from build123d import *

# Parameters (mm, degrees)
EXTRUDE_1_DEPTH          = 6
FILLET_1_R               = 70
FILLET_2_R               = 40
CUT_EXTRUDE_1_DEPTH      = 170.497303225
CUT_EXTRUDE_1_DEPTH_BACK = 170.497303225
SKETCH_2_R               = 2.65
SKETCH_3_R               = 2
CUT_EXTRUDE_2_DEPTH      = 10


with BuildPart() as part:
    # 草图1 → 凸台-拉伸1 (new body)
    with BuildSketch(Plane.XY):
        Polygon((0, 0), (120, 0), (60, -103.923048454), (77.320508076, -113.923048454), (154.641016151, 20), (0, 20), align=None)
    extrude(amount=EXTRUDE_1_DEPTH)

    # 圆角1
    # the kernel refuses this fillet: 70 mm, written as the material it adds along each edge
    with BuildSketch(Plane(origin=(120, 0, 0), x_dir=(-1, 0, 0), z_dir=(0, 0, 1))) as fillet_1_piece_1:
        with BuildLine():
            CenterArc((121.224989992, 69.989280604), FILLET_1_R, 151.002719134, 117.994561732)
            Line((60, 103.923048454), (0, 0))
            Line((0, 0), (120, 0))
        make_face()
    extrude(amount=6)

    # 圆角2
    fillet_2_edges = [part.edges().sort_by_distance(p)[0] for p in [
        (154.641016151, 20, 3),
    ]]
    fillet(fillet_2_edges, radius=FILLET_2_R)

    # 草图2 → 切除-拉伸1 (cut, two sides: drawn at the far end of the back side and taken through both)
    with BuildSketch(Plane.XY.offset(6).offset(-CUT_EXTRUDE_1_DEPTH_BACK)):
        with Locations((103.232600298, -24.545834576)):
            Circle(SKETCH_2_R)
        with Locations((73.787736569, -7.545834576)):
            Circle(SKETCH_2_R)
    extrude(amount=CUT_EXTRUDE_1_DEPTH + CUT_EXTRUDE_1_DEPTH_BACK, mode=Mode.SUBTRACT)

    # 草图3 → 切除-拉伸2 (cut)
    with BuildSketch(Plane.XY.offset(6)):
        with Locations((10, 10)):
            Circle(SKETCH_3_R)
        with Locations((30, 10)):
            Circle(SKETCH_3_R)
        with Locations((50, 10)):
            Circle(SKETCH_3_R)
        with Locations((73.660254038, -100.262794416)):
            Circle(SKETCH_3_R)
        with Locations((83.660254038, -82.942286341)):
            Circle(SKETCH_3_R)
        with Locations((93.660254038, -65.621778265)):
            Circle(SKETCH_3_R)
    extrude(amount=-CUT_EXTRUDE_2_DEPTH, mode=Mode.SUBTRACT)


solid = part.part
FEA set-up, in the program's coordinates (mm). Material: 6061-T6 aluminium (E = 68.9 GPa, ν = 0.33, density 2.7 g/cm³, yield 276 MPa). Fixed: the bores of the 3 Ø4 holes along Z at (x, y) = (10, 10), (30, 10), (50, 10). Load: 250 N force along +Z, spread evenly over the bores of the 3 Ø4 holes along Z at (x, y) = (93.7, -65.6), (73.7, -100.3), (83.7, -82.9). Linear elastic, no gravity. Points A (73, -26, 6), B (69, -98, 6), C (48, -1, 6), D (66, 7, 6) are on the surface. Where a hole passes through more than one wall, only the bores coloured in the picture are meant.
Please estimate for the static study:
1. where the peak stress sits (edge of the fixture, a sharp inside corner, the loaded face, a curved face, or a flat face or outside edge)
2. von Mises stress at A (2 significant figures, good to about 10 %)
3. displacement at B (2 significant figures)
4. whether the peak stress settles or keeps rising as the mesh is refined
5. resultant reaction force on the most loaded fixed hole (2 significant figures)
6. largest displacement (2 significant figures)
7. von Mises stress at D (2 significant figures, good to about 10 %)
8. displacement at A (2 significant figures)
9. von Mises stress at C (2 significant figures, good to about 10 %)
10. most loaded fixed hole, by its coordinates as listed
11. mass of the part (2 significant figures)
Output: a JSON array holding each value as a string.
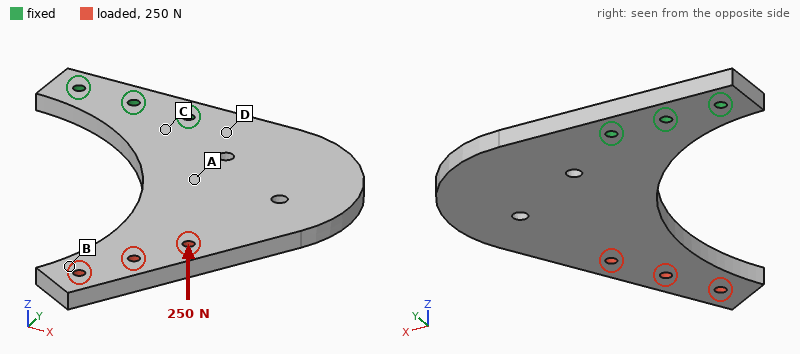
["edge of the fixture", "44 MPa", "1.8 mm", "keeps rising", "470 N", "2.2 mm", "67 MPa", "0.40 mm", "81 MPa", "(50, 10)", "120 g"]
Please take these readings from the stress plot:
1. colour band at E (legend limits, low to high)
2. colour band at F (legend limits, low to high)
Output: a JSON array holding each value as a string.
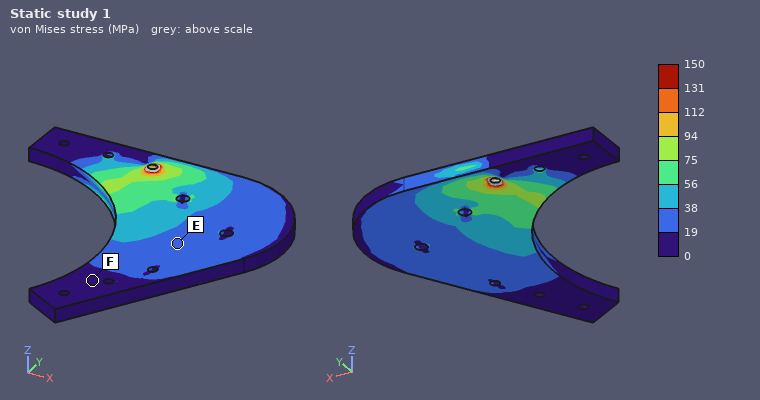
["19 to 38 MPa", "0 to 19 MPa"]
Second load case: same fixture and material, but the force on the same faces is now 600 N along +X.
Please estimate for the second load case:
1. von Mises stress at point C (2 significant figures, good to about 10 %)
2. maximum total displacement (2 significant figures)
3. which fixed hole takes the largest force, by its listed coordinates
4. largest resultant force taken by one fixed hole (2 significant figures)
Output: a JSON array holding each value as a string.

["16 MPa", "0.17 mm", "(50, 10)", "2.0 kN"]
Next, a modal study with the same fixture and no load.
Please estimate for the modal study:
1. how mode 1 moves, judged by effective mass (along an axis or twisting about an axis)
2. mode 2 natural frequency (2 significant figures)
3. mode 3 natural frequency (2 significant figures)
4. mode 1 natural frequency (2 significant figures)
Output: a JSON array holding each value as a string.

["along Z", "810 Hz", "1600 Hz", "360 Hz"]
